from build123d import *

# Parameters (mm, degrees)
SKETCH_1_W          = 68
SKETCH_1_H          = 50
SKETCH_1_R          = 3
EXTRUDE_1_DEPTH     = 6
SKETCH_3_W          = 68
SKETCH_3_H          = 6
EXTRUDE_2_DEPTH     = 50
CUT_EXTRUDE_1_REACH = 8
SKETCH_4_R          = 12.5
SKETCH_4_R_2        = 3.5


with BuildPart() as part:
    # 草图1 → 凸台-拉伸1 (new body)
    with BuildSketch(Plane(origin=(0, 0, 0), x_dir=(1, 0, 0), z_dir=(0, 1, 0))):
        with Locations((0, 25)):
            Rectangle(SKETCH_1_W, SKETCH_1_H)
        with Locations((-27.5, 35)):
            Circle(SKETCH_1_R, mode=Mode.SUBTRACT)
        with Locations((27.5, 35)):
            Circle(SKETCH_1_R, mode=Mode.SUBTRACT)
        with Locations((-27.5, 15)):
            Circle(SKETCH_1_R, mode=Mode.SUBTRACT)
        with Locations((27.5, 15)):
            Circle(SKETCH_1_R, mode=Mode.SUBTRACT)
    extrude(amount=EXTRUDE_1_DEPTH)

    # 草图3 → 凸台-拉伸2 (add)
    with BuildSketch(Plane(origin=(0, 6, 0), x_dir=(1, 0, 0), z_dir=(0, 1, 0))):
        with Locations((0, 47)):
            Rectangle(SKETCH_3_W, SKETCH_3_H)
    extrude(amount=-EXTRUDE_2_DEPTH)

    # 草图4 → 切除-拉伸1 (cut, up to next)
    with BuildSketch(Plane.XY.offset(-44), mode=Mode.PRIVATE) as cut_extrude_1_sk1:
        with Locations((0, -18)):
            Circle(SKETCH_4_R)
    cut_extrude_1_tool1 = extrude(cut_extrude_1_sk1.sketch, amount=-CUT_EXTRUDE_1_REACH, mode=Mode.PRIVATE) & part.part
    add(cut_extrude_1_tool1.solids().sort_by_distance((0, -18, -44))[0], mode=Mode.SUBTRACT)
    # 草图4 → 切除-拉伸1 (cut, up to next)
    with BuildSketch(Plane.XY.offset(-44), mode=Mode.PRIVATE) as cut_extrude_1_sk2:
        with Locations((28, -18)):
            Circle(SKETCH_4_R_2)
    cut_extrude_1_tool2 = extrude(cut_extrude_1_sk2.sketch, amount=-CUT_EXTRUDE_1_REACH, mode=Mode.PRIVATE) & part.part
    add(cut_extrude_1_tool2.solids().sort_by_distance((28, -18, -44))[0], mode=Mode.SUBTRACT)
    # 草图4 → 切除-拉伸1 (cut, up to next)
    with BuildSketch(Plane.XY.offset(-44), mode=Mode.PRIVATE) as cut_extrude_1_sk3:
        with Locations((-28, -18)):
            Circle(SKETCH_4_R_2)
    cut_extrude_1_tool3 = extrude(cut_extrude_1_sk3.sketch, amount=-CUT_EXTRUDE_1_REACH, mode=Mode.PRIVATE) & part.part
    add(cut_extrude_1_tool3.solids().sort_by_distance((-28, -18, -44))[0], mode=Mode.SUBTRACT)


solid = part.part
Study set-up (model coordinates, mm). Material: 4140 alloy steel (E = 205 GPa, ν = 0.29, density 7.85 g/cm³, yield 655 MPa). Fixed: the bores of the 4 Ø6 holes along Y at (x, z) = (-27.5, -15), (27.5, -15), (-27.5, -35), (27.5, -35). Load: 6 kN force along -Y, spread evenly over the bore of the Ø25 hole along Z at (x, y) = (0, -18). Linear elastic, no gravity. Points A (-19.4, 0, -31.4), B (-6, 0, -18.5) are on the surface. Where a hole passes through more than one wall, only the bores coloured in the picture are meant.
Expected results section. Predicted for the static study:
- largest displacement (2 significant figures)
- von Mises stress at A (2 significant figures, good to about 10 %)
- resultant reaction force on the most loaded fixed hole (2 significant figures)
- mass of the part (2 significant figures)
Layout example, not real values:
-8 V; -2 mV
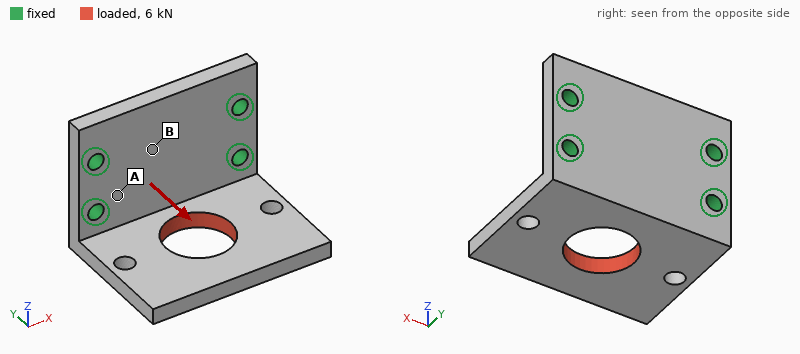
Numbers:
100 µm; 57 MPa; 3.5 kN; 270 g
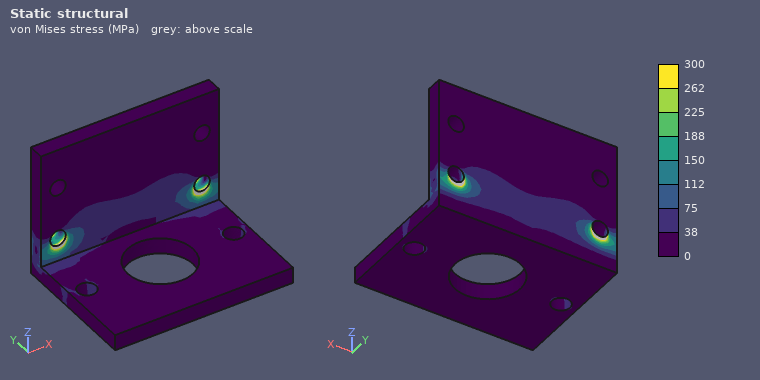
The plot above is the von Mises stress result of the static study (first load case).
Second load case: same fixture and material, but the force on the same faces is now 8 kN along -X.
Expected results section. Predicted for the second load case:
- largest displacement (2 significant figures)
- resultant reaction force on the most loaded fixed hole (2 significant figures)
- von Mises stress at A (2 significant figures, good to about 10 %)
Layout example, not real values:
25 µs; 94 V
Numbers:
65 µm; 4.8 kN; 29 MPa
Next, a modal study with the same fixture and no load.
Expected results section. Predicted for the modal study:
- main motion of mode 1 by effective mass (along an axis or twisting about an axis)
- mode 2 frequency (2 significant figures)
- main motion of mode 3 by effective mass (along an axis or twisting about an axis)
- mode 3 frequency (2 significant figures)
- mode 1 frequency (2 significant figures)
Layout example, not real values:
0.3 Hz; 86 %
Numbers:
along Z; 3200 Hz; along X; 6100 Hz; 1500 Hz
